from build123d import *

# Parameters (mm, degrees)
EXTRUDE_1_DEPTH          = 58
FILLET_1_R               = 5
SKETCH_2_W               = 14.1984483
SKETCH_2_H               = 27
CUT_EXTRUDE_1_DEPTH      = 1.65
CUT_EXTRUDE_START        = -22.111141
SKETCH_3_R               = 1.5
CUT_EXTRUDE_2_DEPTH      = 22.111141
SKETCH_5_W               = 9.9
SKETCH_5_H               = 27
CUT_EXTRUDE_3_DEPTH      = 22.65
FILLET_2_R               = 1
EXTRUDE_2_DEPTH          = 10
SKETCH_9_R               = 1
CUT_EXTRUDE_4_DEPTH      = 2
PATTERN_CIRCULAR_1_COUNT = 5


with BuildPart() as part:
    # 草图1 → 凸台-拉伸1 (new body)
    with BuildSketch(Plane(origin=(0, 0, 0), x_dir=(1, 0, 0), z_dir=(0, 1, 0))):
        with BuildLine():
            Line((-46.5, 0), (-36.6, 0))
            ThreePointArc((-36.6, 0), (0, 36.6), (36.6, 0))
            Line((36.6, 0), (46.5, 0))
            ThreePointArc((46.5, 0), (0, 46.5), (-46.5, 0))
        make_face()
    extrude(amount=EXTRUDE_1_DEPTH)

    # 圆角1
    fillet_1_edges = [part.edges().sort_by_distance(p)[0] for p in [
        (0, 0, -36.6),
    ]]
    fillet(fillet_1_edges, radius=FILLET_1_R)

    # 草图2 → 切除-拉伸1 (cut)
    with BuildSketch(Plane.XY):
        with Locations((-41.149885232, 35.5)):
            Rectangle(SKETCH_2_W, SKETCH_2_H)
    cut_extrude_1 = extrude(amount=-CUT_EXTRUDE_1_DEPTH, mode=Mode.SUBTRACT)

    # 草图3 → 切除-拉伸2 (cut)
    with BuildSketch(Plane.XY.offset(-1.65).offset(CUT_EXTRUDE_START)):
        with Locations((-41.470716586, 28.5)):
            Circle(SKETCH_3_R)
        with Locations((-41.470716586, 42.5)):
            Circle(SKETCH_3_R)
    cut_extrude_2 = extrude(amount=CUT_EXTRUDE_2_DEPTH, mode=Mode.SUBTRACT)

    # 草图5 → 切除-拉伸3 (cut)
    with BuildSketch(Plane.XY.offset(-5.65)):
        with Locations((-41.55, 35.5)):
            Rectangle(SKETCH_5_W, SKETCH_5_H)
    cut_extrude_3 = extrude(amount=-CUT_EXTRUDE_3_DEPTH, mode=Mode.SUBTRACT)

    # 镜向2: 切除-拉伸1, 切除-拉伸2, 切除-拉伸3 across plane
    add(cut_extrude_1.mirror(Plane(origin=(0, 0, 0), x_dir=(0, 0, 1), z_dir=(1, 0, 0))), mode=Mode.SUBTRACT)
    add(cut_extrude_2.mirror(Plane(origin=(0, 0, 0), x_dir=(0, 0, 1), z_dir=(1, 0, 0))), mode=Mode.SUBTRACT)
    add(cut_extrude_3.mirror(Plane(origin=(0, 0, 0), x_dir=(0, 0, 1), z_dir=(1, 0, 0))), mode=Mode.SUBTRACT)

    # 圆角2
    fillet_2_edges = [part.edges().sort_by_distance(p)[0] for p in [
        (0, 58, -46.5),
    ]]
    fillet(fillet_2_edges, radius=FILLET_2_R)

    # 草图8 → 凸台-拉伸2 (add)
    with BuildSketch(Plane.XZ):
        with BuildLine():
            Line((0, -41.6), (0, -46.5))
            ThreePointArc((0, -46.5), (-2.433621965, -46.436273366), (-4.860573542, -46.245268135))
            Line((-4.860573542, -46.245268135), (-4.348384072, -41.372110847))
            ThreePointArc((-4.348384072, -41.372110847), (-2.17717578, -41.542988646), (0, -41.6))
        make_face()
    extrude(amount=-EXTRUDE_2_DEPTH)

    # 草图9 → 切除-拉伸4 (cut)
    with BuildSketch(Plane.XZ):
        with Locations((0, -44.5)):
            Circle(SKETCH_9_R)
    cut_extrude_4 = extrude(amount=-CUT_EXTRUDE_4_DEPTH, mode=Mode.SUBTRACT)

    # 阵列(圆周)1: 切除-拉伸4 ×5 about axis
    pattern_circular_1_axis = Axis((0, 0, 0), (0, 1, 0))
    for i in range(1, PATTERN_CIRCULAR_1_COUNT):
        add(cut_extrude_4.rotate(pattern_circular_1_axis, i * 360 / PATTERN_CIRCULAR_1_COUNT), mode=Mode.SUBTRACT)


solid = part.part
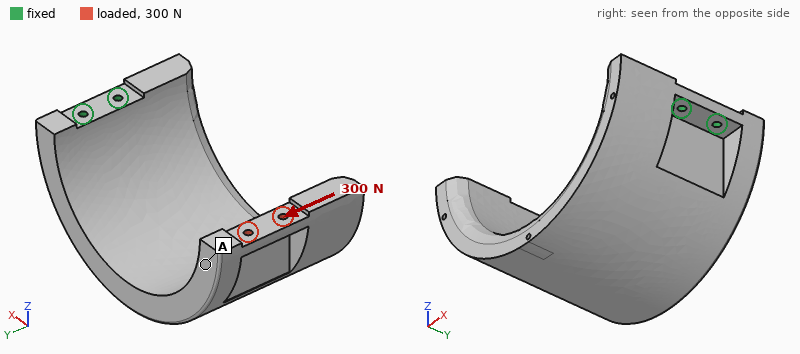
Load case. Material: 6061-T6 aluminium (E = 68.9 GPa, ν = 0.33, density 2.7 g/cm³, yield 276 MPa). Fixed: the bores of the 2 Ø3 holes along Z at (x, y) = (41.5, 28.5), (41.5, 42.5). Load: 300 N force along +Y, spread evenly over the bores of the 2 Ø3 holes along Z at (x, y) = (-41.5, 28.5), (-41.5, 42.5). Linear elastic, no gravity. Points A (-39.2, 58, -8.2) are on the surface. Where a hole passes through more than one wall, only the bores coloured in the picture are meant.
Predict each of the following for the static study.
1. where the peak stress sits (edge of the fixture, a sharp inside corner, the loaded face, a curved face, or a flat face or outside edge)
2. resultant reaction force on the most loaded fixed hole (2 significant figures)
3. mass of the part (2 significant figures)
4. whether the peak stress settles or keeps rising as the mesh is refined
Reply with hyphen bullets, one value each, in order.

- edge of the fixture
- 1.2 kN
- 180 g
- keeps rising
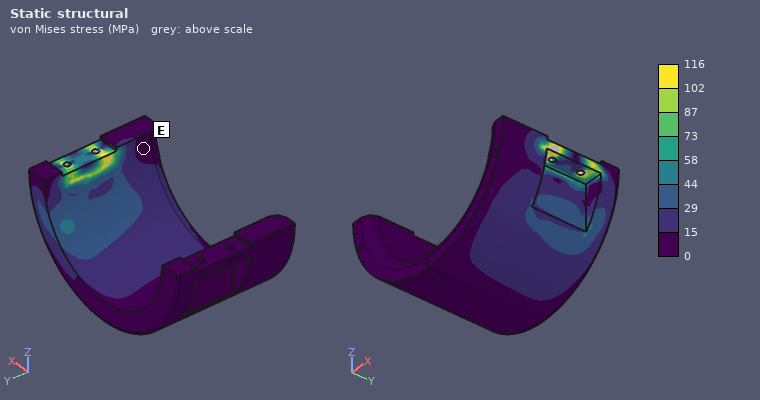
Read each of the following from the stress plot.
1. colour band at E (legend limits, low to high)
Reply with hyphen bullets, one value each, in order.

- 0 to 15 MPa
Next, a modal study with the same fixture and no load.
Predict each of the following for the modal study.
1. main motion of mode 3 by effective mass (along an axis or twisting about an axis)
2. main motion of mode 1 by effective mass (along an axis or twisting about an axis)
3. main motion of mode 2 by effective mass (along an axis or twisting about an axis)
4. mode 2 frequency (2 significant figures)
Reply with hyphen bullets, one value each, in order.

- along Y
- along Z
- along Y
- 540 Hz
